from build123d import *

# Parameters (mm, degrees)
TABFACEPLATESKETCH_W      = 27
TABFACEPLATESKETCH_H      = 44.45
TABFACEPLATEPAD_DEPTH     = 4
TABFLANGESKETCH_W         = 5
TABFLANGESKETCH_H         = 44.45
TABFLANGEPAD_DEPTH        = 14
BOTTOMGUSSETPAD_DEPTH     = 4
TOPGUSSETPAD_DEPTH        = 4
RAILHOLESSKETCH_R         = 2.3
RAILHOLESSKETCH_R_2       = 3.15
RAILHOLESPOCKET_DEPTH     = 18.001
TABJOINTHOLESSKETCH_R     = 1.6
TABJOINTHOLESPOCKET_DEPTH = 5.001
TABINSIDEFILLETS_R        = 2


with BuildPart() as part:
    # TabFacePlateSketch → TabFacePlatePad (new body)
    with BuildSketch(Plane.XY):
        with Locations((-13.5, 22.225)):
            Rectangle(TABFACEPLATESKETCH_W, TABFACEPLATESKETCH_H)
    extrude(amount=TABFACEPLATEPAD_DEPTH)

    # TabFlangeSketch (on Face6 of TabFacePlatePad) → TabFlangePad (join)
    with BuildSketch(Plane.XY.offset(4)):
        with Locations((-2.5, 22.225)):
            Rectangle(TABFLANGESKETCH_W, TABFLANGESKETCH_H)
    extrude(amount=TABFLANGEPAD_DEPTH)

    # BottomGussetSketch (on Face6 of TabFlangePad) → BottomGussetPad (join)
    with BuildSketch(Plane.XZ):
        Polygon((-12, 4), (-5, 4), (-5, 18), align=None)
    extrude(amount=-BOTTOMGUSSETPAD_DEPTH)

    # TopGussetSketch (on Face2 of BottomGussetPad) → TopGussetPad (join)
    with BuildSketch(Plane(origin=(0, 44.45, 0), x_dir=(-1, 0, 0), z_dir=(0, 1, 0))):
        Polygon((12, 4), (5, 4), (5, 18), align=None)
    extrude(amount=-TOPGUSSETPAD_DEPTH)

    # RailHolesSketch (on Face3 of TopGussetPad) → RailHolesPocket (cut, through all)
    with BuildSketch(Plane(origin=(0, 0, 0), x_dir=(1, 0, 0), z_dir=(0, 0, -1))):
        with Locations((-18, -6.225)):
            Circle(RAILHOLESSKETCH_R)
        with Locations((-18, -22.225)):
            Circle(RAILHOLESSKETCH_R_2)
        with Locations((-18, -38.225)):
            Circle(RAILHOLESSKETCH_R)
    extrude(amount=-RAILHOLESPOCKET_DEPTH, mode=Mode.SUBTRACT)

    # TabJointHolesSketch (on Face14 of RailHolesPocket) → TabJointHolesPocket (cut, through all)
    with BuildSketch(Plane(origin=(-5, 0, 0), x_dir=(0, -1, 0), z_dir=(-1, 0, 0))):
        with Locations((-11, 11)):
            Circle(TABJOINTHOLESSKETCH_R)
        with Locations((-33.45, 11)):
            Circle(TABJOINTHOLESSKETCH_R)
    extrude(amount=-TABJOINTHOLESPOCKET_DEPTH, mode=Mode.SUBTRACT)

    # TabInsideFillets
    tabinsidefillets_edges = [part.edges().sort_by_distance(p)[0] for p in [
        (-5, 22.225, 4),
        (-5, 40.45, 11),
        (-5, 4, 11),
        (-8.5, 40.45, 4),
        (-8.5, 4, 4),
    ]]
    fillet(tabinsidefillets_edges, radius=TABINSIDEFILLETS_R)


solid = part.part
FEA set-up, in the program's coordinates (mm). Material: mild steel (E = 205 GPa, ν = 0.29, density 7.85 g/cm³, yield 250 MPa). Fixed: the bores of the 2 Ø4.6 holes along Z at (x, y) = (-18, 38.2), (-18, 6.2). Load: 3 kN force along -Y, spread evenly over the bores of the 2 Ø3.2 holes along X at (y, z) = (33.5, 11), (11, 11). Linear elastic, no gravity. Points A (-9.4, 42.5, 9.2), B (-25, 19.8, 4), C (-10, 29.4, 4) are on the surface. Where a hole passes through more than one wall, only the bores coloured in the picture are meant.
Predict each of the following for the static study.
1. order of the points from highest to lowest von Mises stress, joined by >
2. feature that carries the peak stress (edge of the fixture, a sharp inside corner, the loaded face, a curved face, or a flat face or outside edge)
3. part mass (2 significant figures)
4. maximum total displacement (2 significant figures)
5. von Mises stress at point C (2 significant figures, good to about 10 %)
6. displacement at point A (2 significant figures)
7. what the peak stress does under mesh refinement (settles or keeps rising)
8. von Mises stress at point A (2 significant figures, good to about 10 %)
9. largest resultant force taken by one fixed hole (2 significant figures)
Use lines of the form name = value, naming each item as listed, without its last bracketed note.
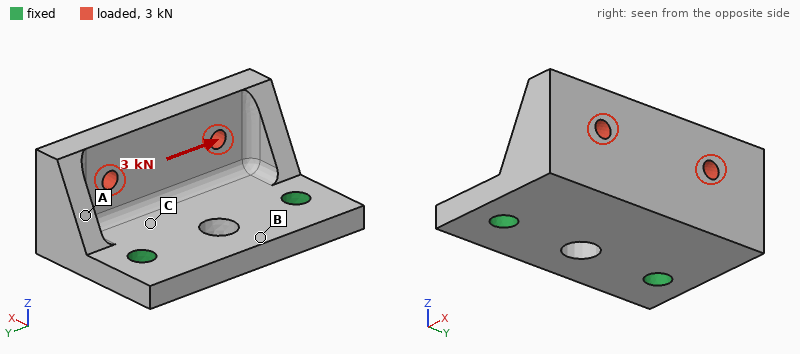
order of the points from highest to lowest von Mises stress, joined by > = C > A > B
feature that carries the peak stress = edge of the fixture
part mass = 63 g
maximum total displacement = 34 µm
von Mises stress at point C = 72 MPa
displacement at point A = 17 µm
what the peak stress does under mesh refinement = keeps rising
von Mises stress at point A = 44 MPa
largest resultant force taken by one fixed hole = 2.1 kN
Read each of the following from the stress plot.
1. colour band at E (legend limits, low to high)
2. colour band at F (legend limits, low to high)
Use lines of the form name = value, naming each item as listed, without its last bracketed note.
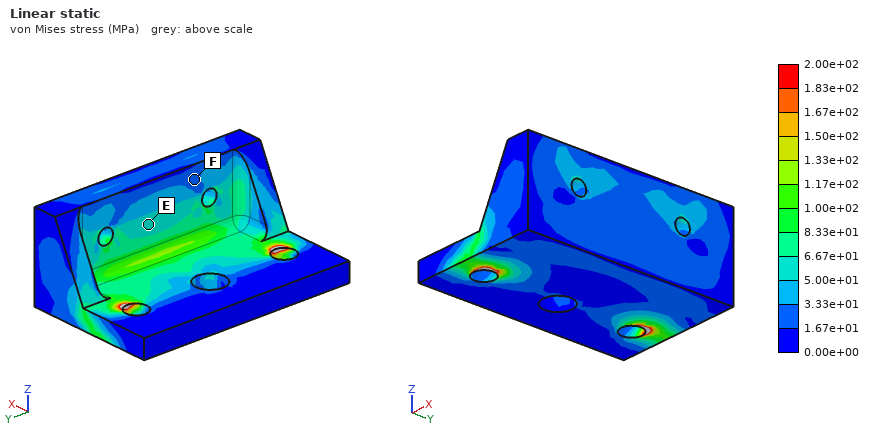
colour band at E = 5.00e+01 to 6.67e+01 MPa
colour band at F = 1.67e+01 to 3.33e+01 MPa
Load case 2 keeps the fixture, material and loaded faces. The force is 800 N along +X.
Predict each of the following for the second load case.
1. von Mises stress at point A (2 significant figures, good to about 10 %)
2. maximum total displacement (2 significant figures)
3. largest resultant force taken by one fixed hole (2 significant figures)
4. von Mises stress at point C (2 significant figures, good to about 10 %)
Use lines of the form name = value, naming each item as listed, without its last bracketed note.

von Mises stress at point A = 17 MPa
maximum total displacement = 37 µm
largest resultant force taken by one fixed hole = 410 N
von Mises stress at point C = 44 MPa
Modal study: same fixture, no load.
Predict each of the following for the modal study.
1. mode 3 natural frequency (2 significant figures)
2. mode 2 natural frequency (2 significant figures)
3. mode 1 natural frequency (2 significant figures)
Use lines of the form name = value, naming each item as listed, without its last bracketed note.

mode 3 natural frequency = 16 kHz
mode 2 natural frequency = 7900 Hz
mode 1 natural frequency = 4100 Hz
